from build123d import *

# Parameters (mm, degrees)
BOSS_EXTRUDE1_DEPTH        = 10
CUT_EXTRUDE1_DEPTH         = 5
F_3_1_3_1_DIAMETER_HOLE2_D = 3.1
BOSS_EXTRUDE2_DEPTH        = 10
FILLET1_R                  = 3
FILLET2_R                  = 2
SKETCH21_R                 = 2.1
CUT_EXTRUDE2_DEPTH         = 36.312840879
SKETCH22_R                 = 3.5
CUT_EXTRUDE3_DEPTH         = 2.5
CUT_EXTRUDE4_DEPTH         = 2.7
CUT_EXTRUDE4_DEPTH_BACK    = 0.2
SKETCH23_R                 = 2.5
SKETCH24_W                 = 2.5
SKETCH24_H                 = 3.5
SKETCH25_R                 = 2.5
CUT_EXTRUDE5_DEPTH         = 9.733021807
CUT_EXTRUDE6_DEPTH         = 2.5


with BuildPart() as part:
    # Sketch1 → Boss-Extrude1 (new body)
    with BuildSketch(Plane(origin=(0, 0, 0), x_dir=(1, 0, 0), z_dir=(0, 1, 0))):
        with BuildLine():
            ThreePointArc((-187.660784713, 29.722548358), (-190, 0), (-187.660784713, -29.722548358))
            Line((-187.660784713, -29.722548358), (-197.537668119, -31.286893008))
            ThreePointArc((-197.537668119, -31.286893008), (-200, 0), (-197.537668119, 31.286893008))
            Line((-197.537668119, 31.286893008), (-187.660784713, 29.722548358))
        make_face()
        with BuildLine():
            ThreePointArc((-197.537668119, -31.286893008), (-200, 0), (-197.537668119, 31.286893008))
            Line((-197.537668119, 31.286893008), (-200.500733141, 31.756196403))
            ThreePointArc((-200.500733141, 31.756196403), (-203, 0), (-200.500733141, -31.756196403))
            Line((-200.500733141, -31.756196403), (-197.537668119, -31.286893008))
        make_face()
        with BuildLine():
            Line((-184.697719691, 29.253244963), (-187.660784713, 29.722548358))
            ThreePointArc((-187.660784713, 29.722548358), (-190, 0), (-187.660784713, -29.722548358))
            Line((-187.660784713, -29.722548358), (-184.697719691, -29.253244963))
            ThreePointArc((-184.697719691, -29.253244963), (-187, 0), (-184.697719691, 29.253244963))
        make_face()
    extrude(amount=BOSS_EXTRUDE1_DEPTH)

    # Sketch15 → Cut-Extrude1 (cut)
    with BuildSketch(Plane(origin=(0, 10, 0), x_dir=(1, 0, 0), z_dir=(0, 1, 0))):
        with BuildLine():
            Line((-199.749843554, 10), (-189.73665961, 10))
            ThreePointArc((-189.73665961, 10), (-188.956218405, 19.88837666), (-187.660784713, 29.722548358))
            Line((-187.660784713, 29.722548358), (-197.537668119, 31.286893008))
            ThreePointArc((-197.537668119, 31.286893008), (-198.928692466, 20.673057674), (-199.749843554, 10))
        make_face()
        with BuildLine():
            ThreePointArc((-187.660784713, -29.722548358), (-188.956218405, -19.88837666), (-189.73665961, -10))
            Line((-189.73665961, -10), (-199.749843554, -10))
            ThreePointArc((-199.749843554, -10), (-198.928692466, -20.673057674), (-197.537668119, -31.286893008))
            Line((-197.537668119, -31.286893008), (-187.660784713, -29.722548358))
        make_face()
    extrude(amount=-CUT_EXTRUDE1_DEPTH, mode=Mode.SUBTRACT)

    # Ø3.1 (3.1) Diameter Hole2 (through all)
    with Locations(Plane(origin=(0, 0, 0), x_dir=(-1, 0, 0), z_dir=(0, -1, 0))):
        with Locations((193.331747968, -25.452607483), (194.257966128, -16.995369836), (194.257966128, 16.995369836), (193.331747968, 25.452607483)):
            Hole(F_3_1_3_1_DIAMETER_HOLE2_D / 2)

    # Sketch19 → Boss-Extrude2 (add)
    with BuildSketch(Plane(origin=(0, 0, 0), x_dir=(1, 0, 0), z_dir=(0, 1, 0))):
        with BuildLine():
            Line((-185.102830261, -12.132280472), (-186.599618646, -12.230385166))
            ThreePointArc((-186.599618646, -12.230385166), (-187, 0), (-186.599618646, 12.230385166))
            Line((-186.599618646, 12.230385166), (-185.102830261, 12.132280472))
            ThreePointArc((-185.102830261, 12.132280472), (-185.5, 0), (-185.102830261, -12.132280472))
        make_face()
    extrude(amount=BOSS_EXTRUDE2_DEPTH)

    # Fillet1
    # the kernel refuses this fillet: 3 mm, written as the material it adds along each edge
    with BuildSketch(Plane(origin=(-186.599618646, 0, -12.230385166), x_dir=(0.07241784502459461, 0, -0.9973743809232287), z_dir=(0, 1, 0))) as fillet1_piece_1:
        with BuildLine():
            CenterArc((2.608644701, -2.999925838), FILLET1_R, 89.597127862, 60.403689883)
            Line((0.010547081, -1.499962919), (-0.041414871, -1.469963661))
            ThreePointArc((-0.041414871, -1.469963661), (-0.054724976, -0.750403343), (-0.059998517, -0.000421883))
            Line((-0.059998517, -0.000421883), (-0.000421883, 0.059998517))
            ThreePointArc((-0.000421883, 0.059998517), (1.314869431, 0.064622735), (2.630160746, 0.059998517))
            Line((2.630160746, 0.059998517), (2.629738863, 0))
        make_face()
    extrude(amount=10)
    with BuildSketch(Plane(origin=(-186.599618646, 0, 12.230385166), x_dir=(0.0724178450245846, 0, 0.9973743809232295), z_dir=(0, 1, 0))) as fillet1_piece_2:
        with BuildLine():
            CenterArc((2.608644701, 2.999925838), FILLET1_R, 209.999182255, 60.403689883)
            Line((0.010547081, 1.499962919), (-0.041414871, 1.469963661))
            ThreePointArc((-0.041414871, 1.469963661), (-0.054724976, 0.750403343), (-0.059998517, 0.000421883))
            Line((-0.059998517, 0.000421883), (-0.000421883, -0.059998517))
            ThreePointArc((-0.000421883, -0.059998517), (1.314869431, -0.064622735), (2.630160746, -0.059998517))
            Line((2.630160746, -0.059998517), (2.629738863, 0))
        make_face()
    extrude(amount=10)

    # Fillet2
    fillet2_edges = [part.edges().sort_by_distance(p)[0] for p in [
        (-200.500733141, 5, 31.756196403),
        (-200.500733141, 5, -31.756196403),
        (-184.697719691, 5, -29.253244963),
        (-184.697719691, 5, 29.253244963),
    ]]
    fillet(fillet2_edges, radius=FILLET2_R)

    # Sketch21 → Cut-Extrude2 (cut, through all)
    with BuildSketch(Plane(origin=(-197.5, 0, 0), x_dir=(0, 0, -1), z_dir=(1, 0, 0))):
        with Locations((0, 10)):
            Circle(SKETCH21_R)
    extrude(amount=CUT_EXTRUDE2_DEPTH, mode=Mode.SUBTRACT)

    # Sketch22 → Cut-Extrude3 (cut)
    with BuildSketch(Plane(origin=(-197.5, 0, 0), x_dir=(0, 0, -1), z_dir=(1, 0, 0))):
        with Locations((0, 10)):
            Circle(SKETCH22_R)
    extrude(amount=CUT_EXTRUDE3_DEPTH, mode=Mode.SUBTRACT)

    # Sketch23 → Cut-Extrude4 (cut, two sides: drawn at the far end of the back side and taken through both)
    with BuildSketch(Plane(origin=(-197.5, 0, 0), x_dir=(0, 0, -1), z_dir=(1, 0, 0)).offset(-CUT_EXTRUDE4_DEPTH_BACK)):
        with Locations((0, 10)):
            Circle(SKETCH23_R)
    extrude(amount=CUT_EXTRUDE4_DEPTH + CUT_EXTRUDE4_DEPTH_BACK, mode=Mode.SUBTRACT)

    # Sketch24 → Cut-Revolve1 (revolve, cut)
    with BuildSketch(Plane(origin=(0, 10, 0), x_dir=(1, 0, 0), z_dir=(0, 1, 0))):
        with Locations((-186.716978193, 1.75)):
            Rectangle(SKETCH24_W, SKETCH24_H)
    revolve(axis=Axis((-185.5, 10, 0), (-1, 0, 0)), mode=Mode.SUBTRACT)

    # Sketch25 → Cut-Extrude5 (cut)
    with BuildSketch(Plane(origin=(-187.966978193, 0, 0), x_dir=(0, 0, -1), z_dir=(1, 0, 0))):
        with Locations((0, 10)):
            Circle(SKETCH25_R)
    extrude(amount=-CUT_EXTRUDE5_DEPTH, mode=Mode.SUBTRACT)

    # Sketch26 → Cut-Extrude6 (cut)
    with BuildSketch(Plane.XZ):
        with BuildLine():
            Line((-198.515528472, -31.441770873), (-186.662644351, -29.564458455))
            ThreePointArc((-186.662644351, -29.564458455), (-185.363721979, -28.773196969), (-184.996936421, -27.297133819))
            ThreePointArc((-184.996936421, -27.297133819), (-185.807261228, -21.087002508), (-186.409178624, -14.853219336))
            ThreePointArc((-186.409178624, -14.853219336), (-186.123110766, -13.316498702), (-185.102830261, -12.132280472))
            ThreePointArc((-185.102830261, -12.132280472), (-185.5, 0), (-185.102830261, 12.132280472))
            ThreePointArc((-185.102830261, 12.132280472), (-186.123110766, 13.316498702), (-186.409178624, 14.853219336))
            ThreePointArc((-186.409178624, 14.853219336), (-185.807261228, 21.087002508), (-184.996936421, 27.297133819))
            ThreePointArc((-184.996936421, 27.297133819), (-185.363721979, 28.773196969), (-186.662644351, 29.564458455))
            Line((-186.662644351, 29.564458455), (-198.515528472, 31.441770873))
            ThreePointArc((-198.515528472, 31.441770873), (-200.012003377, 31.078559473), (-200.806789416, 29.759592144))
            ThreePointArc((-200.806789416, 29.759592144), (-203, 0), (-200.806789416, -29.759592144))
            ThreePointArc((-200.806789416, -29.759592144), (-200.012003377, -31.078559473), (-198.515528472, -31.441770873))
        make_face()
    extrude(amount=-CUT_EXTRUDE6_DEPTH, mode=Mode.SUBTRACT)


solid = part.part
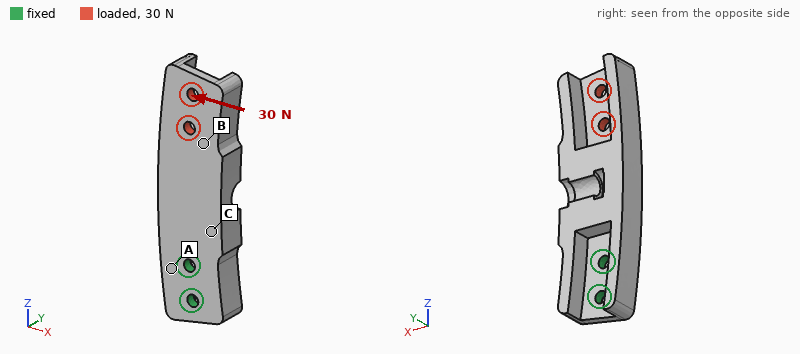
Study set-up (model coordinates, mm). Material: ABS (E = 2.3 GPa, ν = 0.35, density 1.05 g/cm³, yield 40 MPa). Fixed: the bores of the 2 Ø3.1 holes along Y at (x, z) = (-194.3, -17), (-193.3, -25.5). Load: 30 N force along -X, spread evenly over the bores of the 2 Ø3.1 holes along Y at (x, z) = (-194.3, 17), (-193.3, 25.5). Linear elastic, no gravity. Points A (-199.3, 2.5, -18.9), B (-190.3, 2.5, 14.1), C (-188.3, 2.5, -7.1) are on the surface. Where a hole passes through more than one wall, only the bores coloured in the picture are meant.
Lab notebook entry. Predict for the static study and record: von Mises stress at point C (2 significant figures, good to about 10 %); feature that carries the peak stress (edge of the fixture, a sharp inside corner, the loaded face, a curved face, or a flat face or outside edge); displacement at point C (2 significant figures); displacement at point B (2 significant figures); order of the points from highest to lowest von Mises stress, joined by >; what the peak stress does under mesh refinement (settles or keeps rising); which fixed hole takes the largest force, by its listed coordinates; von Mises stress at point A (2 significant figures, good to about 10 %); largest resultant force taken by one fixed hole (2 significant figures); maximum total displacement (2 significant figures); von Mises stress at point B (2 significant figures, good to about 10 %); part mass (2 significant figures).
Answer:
2.3 MPa
edge of the fixture
0.075 mm
0.23 mm
A > C > B
keeps rising
(-194.3, -17)
3.8 MPa
120 N
0.39 mm
1.1 MPa
5.6 g
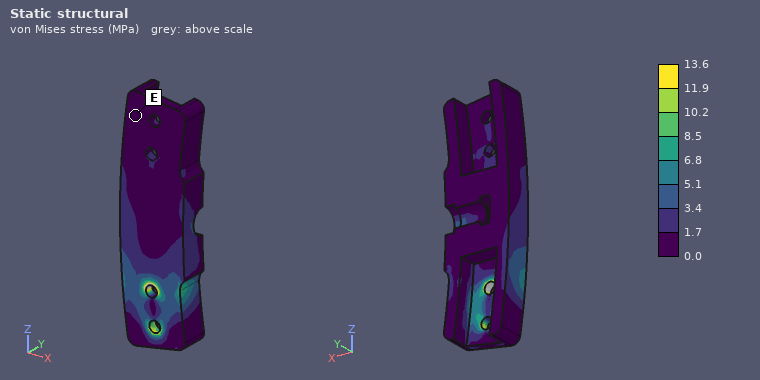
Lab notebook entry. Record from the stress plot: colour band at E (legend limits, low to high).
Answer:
0.0 to 1.7 MPa
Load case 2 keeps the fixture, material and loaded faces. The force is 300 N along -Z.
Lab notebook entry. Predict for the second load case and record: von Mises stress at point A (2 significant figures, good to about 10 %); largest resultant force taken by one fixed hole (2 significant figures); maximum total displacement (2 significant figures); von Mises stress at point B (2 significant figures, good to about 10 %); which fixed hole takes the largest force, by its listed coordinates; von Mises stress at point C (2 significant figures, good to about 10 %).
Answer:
3.9 MPa
230 N
0.63 mm
8.9 MPa
(-194.3, -17)
7.2 MPa
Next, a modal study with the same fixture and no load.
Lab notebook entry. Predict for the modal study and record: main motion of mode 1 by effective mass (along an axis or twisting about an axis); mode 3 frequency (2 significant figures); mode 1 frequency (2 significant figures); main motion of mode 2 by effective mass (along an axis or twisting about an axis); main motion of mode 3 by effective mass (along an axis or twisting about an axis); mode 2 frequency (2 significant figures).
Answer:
along Y
1700 Hz
590 Hz
along X
twisting about Z
1200 Hz
